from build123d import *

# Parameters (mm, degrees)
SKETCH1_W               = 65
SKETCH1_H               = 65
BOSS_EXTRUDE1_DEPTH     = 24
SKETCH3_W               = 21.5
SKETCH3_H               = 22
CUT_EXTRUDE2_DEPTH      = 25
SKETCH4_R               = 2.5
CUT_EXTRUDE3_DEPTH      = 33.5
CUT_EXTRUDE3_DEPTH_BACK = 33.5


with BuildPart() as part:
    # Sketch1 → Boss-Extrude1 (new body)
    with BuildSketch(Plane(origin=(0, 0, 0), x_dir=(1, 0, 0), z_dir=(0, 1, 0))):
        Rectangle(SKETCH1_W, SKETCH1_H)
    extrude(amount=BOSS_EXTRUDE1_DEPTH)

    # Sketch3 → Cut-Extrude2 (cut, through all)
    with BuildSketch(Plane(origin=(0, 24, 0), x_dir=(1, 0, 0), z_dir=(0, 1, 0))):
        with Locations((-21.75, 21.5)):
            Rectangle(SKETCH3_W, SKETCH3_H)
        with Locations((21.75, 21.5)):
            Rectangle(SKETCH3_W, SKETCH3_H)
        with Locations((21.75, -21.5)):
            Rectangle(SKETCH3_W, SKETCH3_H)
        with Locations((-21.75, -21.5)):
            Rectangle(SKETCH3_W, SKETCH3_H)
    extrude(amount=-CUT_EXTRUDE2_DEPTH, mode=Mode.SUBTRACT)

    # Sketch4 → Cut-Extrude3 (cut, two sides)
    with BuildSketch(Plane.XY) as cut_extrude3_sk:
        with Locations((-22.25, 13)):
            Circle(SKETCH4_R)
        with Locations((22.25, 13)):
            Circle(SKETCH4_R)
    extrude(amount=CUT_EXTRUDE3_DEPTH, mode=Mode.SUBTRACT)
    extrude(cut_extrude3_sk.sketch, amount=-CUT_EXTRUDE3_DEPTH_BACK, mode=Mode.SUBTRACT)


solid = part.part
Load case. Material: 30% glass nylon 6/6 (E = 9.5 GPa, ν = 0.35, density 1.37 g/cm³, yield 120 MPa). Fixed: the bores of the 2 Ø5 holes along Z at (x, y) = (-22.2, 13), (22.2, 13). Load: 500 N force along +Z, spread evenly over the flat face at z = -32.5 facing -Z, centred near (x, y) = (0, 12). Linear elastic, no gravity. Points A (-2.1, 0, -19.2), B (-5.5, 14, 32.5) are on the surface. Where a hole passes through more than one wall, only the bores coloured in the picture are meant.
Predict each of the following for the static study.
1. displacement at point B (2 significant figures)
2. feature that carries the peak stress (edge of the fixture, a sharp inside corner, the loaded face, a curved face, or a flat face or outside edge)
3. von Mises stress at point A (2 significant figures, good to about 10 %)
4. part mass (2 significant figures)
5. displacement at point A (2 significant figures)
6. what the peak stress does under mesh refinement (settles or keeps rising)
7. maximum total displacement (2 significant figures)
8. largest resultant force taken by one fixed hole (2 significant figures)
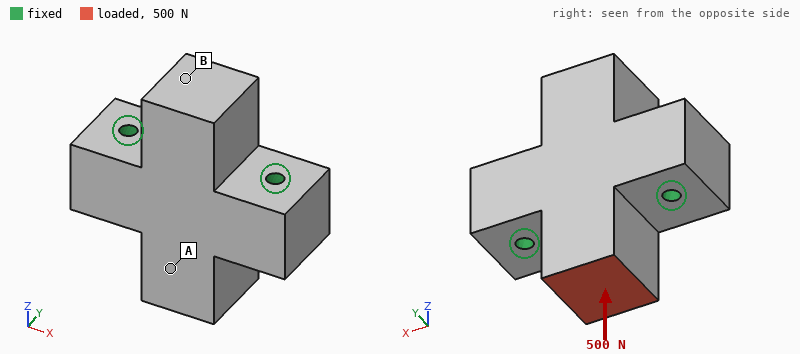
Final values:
2.5 µm
edge of the fixture
0.83 MPa
76 g
4.5 µm
keeps rising
5.8 µm
250 N
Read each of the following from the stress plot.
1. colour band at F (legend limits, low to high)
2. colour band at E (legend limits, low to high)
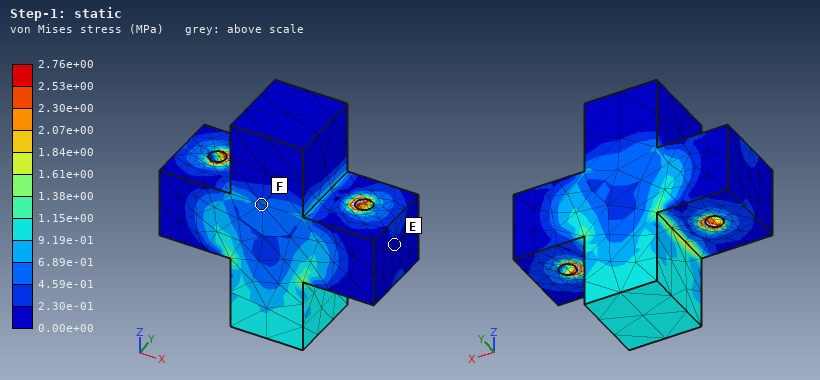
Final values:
4.59e-01 to 6.89e-01 MPa
0.00e+00 to 2.30e-01 MPa
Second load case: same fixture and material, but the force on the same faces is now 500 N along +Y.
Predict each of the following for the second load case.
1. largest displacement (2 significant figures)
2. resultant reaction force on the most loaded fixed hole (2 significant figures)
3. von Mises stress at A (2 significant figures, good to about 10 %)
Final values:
67 µm
250 N
3.1 MPa
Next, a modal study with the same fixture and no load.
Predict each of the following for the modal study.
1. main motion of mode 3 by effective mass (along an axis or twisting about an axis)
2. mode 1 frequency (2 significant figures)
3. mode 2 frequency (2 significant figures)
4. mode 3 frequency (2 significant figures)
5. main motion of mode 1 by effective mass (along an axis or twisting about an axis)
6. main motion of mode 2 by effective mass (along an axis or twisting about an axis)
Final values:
twisting about Y
4300 Hz
5900 Hz
7600 Hz
twisting about X
along Y
